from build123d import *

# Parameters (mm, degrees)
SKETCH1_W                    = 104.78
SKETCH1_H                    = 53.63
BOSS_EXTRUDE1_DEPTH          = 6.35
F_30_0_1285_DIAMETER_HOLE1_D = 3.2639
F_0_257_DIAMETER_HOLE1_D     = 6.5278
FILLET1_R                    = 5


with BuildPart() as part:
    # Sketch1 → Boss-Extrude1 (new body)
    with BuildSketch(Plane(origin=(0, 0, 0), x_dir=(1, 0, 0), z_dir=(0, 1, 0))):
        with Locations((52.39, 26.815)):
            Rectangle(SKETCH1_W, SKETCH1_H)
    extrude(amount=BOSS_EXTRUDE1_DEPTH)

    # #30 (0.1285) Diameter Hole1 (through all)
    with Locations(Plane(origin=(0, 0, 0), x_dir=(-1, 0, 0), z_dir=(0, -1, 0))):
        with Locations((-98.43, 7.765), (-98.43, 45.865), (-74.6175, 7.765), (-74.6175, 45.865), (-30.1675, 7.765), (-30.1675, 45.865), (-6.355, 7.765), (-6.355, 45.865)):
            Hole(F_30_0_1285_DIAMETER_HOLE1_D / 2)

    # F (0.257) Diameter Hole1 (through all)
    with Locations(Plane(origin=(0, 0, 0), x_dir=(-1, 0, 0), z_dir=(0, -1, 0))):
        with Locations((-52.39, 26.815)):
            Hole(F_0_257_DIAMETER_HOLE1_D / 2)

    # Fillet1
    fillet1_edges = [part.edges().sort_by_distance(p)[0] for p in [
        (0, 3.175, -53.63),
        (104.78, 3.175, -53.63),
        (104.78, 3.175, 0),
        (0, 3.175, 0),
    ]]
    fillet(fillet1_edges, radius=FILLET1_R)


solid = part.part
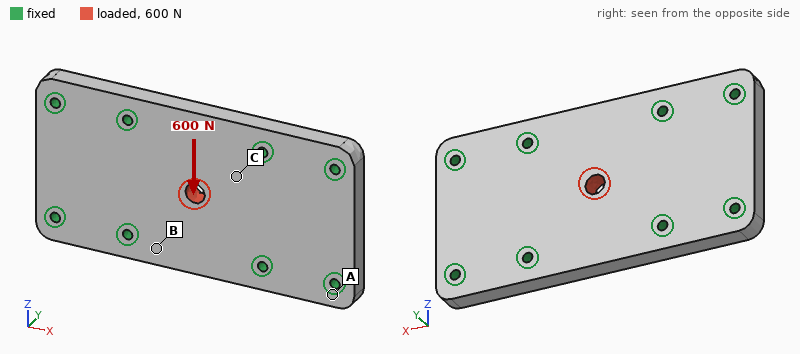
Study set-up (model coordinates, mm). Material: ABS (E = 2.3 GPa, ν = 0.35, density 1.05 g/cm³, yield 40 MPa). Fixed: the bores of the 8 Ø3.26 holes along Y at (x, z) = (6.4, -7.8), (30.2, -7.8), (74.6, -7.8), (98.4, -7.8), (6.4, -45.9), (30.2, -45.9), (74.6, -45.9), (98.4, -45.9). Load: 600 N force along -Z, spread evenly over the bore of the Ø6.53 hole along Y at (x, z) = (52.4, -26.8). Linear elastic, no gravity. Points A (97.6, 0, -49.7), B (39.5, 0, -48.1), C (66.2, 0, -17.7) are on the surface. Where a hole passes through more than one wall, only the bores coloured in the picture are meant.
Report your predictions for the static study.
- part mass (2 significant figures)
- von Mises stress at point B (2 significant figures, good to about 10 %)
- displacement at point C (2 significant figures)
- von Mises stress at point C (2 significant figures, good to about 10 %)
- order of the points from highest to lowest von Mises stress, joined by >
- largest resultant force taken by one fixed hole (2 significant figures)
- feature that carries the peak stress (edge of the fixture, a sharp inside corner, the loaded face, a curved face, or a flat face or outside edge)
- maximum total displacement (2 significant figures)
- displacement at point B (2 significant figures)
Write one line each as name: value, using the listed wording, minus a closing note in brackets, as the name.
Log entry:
part mass: 37 g
von Mises stress at point B: 1.1 MPa
displacement at point C: 14 µm
von Mises stress at point C: 2.0 MPa
order of the points from highest to lowest von Mises stress, joined by >: C > B > A
largest resultant force taken by one fixed hole: 160 N
feature that carries the peak stress: the loaded face
maximum total displacement: 38 µm
displacement at point B: 14 µm
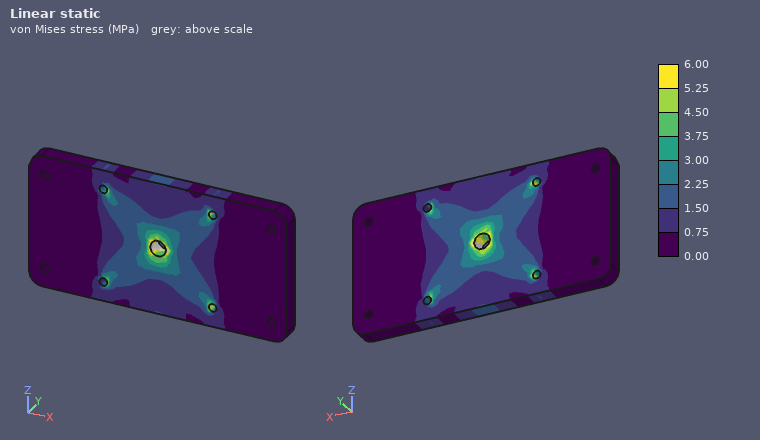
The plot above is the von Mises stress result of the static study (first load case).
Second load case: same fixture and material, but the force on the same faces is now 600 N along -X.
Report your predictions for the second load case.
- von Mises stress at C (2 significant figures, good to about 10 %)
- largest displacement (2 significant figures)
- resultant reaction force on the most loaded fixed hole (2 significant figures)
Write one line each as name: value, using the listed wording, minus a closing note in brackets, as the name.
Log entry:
von Mises stress at C: 1.6 MPa
largest displacement: 28 µm
resultant reaction force on the most loaded fixed hole: 120 N
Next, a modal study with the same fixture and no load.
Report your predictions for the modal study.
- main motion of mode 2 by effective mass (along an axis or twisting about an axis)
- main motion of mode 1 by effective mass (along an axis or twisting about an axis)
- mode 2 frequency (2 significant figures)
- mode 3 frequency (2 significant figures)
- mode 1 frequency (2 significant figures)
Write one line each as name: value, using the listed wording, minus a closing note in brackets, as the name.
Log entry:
main motion of mode 2 by effective mass: twisting about X
main motion of mode 1 by effective mass: along Y
mode 2 frequency: 4600 Hz
mode 3 frequency: 5100 Hz
mode 1 frequency: 3400 Hz
